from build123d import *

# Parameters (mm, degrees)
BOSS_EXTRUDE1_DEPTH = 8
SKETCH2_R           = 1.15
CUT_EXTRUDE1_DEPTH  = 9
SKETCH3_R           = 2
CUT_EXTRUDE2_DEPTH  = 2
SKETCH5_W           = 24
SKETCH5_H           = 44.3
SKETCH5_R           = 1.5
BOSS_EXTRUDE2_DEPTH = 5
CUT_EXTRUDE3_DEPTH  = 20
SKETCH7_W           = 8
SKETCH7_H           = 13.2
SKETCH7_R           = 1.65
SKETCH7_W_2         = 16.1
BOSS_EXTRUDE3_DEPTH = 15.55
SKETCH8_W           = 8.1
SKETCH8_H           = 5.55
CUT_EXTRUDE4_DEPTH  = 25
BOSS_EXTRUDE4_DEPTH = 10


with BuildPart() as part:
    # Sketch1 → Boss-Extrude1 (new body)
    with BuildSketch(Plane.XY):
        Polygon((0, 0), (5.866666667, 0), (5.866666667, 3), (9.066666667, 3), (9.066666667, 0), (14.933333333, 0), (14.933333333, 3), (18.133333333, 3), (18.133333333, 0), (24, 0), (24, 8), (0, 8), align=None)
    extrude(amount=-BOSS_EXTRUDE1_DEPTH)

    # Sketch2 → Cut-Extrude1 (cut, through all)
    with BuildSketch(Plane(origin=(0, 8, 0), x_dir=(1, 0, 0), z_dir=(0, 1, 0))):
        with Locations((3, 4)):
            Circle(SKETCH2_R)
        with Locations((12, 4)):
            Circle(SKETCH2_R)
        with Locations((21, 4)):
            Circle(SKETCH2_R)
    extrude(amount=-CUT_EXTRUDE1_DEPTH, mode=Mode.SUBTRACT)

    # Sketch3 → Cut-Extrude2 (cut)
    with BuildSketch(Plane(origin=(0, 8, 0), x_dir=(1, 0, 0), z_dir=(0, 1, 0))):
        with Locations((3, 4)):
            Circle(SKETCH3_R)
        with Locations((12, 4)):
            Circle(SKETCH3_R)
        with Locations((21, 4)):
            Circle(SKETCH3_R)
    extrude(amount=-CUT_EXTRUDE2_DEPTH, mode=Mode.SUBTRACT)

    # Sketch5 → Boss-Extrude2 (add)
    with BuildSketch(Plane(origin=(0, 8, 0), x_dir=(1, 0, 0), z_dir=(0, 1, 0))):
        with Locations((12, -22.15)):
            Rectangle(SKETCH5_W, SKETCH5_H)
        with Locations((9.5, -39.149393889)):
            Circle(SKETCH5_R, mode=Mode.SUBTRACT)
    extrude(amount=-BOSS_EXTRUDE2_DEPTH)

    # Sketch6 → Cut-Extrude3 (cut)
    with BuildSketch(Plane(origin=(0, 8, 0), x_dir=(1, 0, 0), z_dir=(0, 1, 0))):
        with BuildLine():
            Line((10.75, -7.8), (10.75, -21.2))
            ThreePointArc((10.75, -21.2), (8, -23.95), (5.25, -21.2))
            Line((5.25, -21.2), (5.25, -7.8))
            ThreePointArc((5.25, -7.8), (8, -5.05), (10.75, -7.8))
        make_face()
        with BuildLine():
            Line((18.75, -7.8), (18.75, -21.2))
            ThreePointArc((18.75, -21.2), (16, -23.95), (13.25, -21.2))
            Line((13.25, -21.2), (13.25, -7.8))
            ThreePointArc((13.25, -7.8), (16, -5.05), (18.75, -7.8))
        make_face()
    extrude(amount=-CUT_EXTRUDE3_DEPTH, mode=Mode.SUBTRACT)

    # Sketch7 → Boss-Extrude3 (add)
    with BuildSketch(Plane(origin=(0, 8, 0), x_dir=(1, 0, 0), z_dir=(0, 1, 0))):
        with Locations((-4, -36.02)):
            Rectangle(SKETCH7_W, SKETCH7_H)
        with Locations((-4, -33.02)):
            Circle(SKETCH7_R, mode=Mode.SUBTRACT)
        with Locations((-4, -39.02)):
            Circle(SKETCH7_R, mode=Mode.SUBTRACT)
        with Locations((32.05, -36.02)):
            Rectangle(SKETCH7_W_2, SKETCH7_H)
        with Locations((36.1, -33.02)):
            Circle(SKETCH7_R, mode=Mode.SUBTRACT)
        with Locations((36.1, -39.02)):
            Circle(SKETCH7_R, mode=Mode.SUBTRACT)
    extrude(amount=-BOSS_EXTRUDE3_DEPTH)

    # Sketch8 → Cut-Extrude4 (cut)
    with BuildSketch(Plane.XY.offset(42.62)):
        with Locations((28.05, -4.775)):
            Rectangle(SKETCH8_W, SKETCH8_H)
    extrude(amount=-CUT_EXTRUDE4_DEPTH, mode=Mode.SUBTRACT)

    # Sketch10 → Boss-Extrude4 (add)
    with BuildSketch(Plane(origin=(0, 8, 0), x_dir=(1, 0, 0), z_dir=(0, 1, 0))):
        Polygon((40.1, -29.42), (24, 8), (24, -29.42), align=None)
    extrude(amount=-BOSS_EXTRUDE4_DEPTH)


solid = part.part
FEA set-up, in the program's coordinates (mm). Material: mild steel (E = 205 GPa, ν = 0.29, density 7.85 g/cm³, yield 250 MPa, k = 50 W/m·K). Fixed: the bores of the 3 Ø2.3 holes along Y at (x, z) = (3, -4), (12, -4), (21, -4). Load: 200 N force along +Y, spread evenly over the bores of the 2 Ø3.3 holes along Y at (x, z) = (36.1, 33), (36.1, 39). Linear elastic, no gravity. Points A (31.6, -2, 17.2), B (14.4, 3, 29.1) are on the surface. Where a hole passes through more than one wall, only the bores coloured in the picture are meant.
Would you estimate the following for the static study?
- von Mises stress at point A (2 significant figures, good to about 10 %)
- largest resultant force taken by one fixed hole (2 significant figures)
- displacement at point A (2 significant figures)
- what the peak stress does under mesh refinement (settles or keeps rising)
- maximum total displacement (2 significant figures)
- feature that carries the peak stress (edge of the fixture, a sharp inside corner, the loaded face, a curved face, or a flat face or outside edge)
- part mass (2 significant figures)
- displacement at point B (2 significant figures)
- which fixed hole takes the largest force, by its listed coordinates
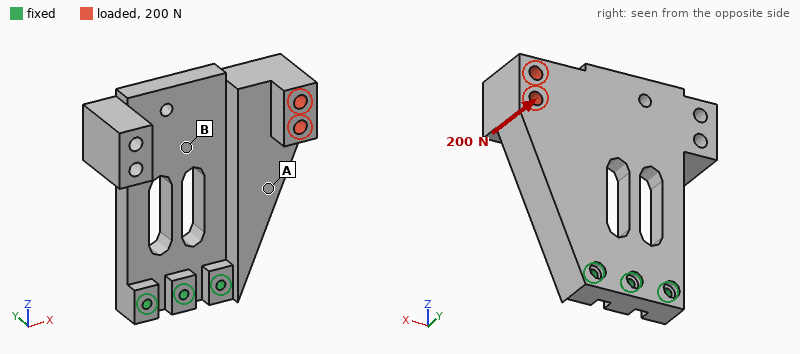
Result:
19 MPa
330 N
29 µm
keeps rising
75 µm
edge of the fixture
97 g
31 µm
(21, -4)
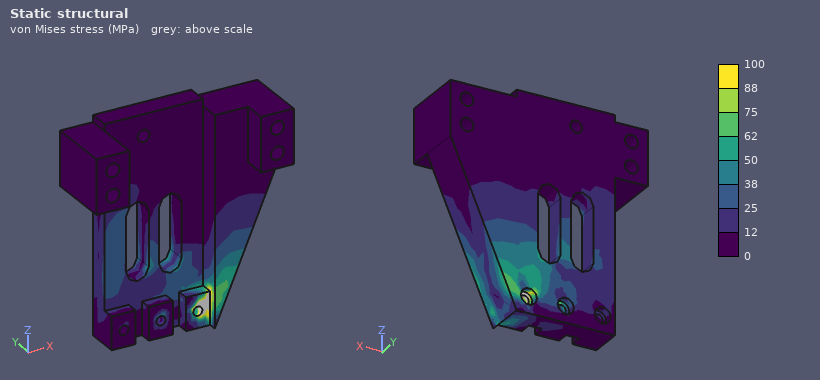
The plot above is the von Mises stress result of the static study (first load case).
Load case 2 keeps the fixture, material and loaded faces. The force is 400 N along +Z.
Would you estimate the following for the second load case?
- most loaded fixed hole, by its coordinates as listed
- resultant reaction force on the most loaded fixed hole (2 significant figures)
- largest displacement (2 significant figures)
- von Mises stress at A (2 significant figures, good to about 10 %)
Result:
(21, -4)
720 N
13 µm
8.7 MPa
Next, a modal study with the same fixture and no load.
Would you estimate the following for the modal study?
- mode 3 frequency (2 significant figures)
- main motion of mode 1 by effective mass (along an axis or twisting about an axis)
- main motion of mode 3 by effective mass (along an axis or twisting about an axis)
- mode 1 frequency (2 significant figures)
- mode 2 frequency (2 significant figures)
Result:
3700 Hz
along Y
along X
1400 Hz
2400 Hz
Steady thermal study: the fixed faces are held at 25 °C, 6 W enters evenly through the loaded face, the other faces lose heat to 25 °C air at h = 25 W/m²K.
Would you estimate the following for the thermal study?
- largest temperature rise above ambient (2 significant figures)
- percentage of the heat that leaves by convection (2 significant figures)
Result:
29 K
35 %
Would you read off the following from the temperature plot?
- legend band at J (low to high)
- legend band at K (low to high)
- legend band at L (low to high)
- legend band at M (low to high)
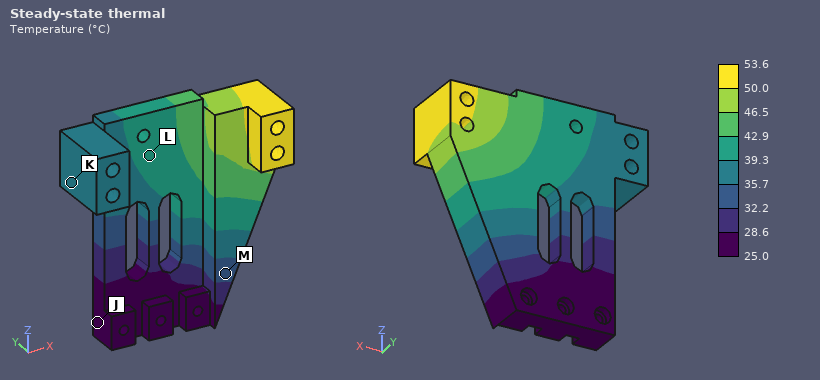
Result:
25.0 to 28.6 °C
35.7 to 39.3 °C
39.3 to 42.9 °C
32.2 to 35.7 °C
